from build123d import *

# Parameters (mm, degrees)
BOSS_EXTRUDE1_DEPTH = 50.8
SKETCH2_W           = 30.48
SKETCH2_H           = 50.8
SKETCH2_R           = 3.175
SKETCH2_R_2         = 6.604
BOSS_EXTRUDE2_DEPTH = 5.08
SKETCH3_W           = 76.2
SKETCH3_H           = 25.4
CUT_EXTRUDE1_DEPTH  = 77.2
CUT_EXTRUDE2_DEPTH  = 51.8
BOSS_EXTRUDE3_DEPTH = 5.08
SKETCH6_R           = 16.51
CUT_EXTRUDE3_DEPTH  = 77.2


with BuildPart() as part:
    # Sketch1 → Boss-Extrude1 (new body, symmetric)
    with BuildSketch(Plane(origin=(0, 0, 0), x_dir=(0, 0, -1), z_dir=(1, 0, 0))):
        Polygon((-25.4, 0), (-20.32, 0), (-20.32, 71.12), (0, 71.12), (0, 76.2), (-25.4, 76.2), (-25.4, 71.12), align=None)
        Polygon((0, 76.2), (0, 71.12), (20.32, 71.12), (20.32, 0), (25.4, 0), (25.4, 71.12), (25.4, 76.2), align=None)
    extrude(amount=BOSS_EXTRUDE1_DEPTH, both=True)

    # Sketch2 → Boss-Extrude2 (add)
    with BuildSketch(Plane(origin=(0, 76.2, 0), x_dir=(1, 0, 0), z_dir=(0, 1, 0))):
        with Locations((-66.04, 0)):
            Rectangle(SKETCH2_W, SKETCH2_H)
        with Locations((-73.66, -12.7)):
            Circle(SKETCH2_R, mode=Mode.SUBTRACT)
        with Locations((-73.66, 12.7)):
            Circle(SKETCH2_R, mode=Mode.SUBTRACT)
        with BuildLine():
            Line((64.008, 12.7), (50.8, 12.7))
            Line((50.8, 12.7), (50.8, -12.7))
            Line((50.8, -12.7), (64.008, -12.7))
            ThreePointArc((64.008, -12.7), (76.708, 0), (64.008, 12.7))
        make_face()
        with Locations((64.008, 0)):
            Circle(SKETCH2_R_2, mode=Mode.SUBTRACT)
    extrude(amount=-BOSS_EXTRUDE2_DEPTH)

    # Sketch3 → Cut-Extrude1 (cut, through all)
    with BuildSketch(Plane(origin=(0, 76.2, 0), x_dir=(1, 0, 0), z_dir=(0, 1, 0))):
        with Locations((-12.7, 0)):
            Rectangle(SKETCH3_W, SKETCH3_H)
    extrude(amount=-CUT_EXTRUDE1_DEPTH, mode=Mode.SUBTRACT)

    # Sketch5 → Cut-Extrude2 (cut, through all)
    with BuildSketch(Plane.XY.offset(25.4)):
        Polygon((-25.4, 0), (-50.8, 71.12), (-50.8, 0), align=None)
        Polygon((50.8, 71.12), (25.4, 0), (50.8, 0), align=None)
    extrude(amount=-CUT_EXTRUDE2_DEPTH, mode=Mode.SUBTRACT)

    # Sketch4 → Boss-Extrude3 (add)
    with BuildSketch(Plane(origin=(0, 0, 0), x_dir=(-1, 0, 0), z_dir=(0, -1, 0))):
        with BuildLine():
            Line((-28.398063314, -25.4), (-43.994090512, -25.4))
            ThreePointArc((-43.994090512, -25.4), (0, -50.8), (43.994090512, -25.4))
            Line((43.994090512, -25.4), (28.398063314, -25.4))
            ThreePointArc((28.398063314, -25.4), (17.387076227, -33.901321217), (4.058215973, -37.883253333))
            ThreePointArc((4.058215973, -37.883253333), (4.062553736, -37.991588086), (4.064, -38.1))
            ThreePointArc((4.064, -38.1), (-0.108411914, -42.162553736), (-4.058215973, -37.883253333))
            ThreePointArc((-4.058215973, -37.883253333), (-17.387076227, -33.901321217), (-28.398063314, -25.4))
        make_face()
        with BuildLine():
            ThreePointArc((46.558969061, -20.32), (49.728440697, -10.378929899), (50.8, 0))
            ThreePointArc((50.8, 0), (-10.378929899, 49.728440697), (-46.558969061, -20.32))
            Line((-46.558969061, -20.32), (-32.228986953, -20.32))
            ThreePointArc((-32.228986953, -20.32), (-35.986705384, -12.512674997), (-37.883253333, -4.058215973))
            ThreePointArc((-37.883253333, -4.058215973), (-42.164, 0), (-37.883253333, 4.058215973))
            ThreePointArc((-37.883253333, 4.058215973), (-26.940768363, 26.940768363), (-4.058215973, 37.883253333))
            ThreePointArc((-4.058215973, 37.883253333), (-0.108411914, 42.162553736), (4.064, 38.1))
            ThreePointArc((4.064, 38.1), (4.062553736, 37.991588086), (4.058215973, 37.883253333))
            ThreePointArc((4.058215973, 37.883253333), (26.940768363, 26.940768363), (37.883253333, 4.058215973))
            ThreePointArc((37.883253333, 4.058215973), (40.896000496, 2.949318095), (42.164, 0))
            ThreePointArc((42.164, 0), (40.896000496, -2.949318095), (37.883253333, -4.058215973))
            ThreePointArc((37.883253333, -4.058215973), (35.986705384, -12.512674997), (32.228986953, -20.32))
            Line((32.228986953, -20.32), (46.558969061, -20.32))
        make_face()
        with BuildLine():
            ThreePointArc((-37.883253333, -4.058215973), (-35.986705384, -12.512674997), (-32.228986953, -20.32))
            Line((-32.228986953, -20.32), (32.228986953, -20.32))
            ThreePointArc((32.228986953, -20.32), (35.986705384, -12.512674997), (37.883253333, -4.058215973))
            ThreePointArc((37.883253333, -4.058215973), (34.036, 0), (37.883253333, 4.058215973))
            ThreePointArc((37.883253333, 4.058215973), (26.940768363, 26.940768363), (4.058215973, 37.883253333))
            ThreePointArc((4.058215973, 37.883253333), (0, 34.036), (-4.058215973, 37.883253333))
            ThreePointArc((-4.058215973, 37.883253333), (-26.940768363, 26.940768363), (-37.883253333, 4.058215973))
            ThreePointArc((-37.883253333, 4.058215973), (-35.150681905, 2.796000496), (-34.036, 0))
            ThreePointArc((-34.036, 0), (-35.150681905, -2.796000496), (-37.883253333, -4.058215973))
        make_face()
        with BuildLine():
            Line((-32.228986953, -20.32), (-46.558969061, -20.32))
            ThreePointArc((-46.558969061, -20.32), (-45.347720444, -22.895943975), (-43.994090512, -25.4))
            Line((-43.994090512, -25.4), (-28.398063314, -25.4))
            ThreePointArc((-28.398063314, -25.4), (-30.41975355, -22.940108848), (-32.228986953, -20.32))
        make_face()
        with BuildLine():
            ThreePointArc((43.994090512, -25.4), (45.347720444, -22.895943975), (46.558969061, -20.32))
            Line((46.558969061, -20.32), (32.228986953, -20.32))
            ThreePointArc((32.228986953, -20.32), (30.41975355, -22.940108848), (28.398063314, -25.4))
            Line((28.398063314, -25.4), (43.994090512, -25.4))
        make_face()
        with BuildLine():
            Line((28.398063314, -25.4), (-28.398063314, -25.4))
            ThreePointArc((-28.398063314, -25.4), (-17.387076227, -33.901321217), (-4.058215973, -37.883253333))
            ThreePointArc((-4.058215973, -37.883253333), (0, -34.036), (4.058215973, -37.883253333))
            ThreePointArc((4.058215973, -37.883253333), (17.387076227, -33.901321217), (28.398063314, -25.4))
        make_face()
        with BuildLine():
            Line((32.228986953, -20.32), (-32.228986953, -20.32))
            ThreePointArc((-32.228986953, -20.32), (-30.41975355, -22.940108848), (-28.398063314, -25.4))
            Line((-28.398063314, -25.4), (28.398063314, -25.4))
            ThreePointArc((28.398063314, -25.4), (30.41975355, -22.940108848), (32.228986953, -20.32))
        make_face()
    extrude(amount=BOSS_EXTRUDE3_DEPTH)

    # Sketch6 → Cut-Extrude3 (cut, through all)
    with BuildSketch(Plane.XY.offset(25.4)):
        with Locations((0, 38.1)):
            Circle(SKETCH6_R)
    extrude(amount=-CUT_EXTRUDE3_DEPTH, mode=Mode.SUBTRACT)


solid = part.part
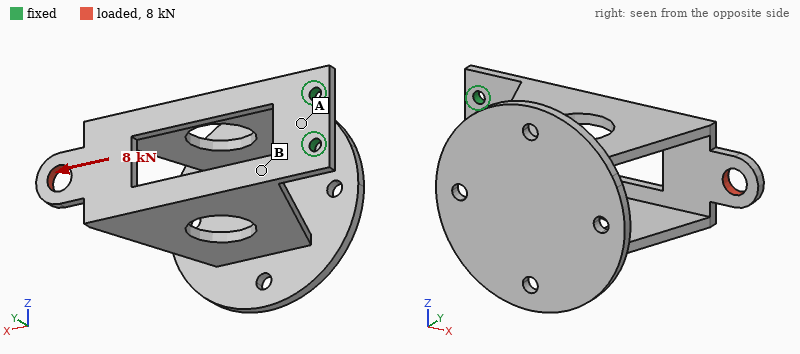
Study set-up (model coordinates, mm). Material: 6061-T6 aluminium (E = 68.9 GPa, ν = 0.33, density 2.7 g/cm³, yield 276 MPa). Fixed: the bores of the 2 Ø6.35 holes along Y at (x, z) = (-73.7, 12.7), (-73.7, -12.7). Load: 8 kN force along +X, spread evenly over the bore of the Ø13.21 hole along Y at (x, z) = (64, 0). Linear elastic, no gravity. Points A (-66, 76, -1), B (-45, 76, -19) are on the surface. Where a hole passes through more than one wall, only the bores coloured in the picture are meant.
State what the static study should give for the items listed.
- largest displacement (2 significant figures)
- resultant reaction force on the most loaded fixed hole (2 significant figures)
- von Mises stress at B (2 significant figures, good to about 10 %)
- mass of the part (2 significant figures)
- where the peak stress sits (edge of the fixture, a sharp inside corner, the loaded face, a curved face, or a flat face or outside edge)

0.29 mm
4.1 kN
69 MPa
300 g
the loaded face
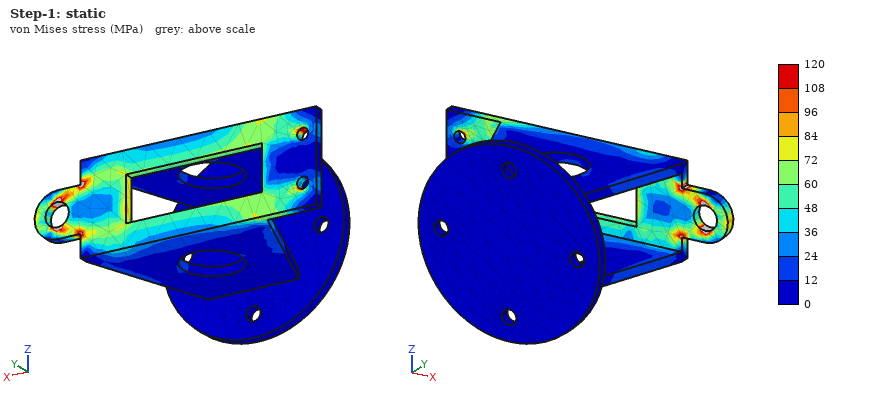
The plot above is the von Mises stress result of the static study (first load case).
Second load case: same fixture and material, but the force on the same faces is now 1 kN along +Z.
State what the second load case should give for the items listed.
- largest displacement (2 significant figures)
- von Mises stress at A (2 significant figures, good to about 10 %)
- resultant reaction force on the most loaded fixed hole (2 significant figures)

0.75 mm
46 MPa
4.5 kN
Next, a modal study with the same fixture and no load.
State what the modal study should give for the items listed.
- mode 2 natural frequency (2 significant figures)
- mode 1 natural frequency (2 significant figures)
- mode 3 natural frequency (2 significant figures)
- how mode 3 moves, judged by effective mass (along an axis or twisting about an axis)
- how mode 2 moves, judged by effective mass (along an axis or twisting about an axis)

260 Hz
110 Hz
700 Hz
along Z
along Z
